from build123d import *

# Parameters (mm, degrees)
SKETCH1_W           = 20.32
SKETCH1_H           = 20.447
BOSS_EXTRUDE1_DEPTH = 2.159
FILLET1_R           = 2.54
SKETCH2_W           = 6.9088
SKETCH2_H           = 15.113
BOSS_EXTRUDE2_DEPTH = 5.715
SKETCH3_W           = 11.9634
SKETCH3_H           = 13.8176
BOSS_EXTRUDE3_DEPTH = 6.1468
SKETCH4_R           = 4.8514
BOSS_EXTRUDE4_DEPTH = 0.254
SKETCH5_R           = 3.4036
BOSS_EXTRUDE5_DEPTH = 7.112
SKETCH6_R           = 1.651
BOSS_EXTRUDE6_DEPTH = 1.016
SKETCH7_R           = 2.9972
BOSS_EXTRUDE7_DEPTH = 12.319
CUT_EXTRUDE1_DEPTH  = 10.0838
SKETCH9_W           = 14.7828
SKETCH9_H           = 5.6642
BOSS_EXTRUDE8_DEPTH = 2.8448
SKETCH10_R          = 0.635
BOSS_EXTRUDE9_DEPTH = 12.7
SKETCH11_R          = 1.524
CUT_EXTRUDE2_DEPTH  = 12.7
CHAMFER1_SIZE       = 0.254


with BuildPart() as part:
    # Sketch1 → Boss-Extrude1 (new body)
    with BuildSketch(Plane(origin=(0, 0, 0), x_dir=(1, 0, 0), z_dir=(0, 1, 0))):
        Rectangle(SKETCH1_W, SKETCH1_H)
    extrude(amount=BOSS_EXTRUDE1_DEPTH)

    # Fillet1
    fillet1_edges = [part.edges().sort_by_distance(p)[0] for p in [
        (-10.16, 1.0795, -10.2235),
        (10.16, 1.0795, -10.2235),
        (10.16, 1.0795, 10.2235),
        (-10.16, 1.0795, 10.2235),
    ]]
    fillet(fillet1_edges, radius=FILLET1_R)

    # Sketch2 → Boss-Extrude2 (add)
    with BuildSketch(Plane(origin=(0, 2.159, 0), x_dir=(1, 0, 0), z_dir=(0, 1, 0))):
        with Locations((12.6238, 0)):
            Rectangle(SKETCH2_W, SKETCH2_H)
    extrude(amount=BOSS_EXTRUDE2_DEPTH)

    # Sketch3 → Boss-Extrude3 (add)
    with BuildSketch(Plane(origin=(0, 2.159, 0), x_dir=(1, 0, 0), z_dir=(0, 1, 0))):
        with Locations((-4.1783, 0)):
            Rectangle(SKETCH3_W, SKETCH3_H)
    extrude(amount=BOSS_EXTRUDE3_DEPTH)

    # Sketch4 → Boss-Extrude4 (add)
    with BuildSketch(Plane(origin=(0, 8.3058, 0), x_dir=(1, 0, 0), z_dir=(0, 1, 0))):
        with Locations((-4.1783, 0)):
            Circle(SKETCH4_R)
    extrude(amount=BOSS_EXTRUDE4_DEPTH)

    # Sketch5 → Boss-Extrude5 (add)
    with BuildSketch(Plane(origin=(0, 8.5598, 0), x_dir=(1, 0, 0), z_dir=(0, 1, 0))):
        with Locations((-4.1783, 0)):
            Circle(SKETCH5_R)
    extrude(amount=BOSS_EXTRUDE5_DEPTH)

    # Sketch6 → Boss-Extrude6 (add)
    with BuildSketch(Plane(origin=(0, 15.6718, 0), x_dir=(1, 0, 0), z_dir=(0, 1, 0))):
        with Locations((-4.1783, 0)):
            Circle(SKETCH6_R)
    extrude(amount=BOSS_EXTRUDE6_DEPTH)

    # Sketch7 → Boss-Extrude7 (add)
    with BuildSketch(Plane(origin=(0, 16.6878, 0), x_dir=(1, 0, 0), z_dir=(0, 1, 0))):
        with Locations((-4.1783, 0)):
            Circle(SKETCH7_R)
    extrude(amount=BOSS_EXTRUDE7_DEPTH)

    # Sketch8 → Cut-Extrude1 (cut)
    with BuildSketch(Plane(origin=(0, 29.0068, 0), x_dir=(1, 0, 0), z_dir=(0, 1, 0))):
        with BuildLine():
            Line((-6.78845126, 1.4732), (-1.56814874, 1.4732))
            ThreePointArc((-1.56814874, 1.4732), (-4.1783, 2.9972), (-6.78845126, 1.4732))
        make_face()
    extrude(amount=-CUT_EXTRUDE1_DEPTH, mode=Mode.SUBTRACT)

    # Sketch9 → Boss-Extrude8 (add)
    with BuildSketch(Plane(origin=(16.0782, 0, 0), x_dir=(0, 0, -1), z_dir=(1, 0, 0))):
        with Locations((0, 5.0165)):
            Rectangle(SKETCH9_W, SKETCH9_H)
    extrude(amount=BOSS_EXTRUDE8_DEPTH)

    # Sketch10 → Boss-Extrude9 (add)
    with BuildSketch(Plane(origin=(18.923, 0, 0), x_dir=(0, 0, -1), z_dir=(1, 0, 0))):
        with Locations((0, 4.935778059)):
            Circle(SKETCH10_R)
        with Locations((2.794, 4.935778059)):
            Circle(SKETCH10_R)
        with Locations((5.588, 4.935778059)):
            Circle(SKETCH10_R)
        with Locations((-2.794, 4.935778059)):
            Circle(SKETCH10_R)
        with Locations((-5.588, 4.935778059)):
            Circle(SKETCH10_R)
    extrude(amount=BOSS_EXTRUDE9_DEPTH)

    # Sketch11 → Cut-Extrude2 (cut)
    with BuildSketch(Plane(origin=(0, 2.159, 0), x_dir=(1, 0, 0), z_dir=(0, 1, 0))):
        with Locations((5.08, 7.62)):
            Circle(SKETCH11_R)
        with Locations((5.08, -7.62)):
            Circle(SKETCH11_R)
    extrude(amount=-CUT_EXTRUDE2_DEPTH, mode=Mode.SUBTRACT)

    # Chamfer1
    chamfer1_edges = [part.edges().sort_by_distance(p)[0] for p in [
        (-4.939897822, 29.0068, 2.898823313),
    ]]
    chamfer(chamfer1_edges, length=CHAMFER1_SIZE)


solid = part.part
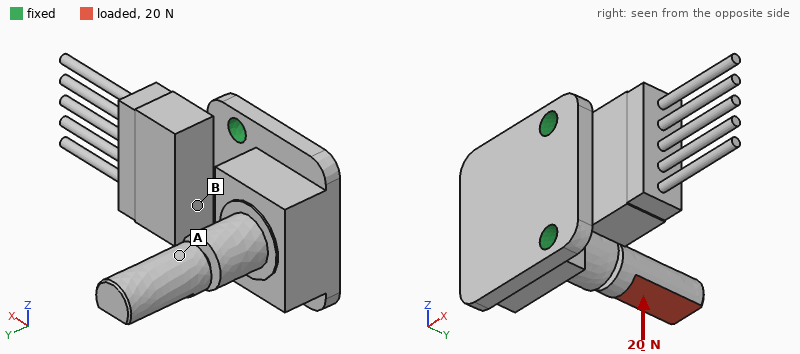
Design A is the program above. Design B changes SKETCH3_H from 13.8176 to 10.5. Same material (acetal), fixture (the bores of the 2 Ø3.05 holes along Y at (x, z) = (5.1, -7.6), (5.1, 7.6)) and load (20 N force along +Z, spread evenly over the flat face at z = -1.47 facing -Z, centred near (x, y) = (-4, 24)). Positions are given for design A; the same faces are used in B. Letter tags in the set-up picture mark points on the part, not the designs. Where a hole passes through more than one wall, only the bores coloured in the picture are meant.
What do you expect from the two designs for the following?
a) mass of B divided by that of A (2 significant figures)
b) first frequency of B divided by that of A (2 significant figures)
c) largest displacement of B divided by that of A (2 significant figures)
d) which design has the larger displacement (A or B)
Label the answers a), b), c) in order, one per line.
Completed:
a) 0.93
b) 0.99
c) 1.1
d) B
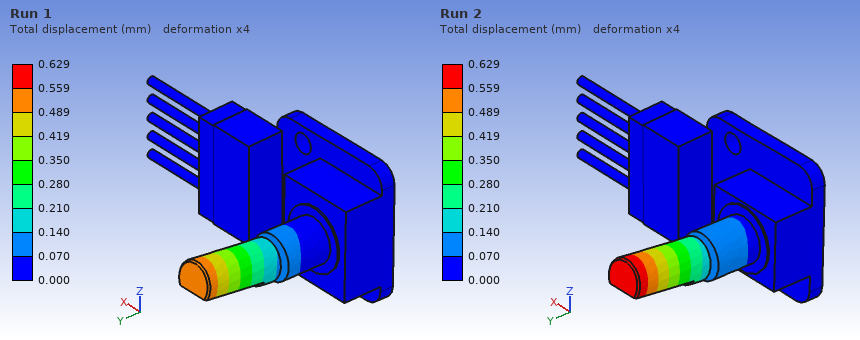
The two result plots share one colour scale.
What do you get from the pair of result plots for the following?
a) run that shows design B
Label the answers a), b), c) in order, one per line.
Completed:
a) Run 2
